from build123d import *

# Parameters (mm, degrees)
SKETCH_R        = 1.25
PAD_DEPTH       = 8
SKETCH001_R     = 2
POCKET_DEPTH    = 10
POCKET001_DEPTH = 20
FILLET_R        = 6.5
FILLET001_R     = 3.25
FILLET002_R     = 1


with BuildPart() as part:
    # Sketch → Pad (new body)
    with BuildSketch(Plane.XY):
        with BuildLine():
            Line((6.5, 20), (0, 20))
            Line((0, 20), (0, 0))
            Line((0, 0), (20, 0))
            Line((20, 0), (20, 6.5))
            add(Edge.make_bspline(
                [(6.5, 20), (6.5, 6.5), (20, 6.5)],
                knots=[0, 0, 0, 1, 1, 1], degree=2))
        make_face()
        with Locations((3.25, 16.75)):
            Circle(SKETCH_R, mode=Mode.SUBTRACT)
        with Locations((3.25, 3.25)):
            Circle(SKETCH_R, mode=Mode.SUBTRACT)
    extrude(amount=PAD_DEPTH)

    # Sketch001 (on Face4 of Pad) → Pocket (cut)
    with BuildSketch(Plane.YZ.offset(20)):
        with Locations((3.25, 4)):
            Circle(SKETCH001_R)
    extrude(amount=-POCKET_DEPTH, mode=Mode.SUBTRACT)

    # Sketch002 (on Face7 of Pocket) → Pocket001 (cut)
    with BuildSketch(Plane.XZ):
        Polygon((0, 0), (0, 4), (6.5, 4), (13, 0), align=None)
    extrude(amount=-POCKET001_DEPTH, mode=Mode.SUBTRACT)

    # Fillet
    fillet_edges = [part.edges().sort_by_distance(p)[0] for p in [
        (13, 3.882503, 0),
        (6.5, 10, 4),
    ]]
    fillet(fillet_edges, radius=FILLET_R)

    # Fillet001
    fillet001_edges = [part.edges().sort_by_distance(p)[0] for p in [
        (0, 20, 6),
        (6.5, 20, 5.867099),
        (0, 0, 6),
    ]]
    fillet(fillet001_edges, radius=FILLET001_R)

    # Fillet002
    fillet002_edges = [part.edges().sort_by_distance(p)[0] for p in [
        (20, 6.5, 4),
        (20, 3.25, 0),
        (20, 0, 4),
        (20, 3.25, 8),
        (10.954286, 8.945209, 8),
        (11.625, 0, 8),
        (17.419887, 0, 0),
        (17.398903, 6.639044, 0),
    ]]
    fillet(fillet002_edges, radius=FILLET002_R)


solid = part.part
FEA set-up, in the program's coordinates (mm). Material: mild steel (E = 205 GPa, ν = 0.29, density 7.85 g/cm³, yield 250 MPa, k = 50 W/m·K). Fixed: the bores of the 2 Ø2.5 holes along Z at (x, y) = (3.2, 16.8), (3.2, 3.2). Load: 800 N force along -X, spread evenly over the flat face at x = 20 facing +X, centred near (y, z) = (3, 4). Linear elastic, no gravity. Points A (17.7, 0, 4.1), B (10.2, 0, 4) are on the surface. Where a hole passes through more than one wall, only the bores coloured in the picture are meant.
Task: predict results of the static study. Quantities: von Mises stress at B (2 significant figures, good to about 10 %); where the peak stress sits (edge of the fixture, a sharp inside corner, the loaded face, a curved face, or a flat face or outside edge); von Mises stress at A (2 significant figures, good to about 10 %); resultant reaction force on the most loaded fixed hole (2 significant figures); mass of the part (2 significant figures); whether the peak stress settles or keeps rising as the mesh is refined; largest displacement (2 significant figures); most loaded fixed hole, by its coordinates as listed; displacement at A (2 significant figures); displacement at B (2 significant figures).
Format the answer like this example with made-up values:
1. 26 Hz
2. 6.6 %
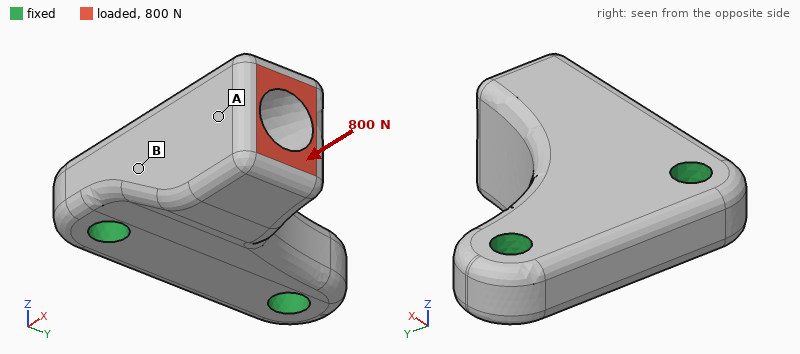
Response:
1. 43 MPa
2. edge of the fixture
3. 16 MPa
4. 780 N
5. 8.5 g
6. keeps rising
7. 13 µm
8. (3.2, 3.2)
9. 9.8 µm
10. 4.0 µm
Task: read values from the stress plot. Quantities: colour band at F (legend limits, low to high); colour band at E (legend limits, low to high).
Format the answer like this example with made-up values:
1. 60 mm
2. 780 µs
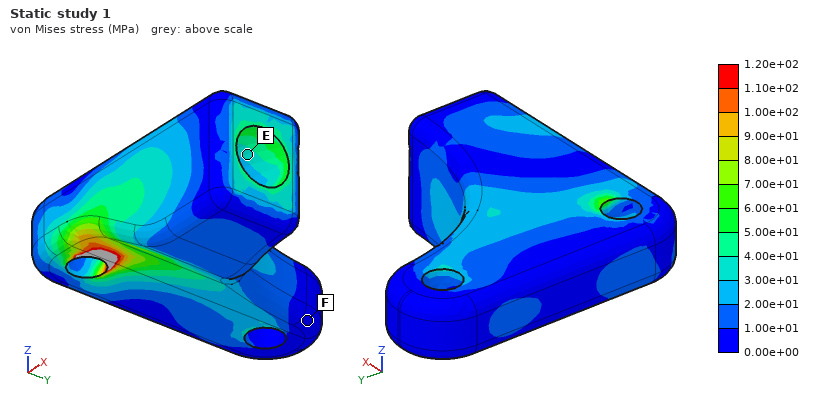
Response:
1. 0.00e+00 to 1.00e+01 MPa
2. 3.00e+01 to 4.00e+01 MPa
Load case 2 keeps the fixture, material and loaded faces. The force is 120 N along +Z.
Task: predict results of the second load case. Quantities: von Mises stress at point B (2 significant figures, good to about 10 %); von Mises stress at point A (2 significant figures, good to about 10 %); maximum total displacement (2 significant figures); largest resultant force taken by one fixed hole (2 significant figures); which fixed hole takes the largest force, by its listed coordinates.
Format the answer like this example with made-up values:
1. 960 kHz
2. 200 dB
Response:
1. 18 MPa
2. 13 MPa
3. 14 µm
4. 120 N
5. (3.2, 3.2)
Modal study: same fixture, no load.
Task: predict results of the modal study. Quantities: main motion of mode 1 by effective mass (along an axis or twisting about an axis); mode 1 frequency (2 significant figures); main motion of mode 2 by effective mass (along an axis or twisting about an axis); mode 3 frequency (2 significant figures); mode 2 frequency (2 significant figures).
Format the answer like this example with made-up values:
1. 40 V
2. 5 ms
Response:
1. along Z
2. 12 kHz
3. along Y
4. 41 kHz
5. 26 kHz
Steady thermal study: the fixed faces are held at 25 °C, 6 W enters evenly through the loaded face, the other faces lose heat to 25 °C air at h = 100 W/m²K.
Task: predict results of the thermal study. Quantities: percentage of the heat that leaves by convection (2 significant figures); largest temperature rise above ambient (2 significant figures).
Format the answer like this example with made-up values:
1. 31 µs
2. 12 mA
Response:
1. 22 %
2. 46 K
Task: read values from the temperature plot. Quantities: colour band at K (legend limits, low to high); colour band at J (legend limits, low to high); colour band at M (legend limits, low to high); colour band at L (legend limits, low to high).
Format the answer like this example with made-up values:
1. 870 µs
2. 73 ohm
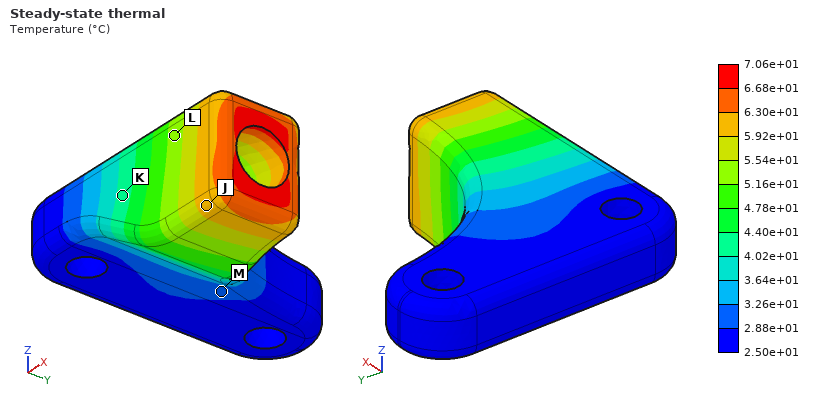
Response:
1. 4.02e+01 to 4.40e+01 °C
2. 5.92e+01 to 6.30e+01 °C
3. 2.88e+01 to 3.26e+01 °C
4. 5.16e+01 to 5.54e+01 °C
